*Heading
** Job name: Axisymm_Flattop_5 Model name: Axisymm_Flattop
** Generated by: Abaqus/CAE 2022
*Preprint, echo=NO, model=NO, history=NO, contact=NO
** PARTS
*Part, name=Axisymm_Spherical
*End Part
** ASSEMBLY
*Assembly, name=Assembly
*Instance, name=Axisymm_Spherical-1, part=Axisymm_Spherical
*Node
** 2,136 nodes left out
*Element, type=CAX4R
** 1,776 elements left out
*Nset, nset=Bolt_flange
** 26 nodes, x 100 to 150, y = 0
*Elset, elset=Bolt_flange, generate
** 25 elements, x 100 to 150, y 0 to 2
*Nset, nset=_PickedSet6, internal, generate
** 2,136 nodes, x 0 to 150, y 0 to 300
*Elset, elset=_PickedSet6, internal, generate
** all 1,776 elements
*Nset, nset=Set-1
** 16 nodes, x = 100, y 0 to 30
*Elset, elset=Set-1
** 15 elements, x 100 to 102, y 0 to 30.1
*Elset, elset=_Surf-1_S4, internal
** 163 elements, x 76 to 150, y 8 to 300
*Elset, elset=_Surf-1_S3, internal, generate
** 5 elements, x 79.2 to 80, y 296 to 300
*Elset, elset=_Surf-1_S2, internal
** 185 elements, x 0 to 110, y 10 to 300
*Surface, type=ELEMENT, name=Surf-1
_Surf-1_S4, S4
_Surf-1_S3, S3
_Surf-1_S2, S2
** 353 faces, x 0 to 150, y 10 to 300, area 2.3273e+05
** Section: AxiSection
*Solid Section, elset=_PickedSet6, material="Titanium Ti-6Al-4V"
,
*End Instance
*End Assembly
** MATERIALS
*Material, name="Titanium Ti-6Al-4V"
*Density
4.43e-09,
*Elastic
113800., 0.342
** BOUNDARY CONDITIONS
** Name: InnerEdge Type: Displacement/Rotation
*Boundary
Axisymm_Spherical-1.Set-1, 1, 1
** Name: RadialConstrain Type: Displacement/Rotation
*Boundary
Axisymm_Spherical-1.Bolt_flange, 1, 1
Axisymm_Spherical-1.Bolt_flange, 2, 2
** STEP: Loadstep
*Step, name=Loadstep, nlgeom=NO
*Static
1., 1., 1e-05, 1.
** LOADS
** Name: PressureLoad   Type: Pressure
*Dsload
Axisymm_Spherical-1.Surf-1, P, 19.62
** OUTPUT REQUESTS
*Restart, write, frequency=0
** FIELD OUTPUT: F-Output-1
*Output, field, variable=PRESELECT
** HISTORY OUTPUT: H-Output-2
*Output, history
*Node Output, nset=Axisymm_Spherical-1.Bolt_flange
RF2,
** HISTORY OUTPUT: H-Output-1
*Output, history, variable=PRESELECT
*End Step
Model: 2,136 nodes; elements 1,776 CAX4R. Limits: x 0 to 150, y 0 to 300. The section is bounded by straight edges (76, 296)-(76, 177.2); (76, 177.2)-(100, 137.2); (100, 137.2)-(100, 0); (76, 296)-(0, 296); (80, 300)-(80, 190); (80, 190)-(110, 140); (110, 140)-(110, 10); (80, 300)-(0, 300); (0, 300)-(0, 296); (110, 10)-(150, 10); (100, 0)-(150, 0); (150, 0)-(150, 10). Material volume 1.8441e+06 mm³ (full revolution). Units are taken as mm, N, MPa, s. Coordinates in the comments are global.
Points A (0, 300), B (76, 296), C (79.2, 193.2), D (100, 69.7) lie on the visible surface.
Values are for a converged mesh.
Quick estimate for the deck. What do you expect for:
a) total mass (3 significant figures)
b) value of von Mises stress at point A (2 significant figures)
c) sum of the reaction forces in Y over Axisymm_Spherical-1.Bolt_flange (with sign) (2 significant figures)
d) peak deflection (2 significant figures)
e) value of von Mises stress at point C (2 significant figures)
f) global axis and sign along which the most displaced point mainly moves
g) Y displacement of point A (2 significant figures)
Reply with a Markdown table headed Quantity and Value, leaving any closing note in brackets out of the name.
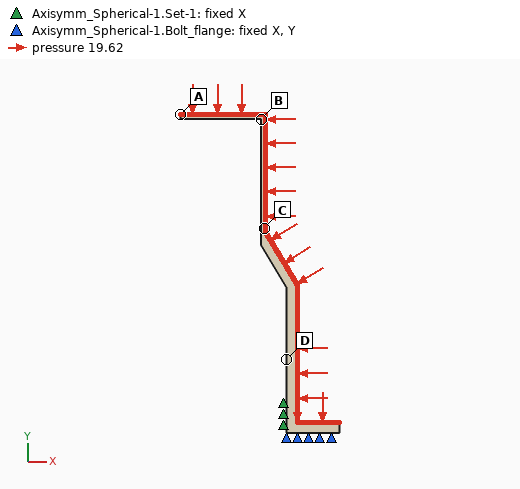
| Quantity | Value |
|---|---|
| total mass | 8.17 kg |
| value of von Mises stress at point A | 4500 MPa |
| sum of the reaction forces in Y over Axisymm_Spherical-1.Bolt_flange (with sign) | 1.4e+06 N |
| peak deflection | 21 mm |
| value of von Mises stress at point C | 450 MPa |
| global axis and sign along which the most displaced point mainly moves | -Y |
| Y displacement of point A | -21 mm |
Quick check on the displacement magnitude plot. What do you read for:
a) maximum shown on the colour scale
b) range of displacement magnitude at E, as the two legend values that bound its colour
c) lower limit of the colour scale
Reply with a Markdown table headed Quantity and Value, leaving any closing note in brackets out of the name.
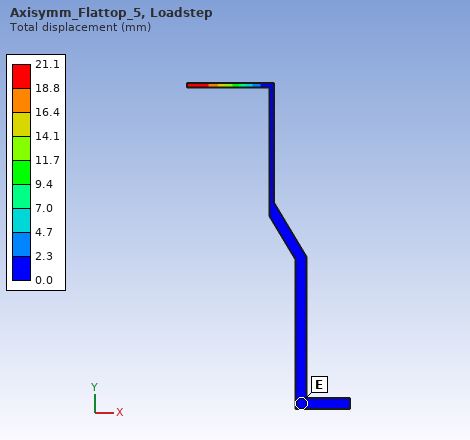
| Quantity | Value |
|---|---|
| maximum shown on the colour scale | 21.1 mm |
| range of displacement magnitude at E, as the two legend values that bound its colour | 0.0 to 2.3 mm |
| lower limit of the colour scale | 0.0 mm |
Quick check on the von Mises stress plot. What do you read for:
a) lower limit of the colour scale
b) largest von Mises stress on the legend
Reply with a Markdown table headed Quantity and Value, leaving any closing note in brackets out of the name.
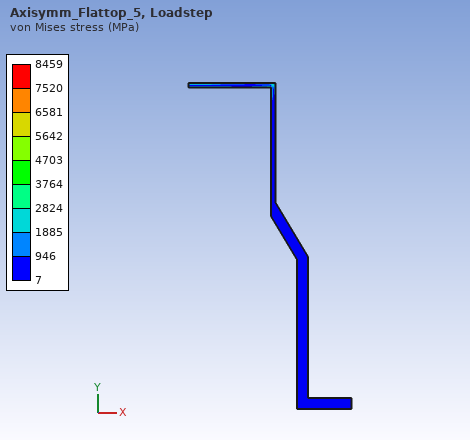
| Quantity | Value |
|---|---|
| lower limit of the colour scale | 7 MPa |
| largest von Mises stress on the legend | 8459 MPa |
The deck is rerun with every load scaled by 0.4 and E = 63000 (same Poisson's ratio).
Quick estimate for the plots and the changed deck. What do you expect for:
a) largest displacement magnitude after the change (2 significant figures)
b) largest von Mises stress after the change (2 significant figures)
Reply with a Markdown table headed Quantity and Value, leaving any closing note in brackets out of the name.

| Quantity | Value |
|---|---|
| largest displacement magnitude after the change | 15 mm |
| largest von Mises stress after the change | 3400 MPa |
